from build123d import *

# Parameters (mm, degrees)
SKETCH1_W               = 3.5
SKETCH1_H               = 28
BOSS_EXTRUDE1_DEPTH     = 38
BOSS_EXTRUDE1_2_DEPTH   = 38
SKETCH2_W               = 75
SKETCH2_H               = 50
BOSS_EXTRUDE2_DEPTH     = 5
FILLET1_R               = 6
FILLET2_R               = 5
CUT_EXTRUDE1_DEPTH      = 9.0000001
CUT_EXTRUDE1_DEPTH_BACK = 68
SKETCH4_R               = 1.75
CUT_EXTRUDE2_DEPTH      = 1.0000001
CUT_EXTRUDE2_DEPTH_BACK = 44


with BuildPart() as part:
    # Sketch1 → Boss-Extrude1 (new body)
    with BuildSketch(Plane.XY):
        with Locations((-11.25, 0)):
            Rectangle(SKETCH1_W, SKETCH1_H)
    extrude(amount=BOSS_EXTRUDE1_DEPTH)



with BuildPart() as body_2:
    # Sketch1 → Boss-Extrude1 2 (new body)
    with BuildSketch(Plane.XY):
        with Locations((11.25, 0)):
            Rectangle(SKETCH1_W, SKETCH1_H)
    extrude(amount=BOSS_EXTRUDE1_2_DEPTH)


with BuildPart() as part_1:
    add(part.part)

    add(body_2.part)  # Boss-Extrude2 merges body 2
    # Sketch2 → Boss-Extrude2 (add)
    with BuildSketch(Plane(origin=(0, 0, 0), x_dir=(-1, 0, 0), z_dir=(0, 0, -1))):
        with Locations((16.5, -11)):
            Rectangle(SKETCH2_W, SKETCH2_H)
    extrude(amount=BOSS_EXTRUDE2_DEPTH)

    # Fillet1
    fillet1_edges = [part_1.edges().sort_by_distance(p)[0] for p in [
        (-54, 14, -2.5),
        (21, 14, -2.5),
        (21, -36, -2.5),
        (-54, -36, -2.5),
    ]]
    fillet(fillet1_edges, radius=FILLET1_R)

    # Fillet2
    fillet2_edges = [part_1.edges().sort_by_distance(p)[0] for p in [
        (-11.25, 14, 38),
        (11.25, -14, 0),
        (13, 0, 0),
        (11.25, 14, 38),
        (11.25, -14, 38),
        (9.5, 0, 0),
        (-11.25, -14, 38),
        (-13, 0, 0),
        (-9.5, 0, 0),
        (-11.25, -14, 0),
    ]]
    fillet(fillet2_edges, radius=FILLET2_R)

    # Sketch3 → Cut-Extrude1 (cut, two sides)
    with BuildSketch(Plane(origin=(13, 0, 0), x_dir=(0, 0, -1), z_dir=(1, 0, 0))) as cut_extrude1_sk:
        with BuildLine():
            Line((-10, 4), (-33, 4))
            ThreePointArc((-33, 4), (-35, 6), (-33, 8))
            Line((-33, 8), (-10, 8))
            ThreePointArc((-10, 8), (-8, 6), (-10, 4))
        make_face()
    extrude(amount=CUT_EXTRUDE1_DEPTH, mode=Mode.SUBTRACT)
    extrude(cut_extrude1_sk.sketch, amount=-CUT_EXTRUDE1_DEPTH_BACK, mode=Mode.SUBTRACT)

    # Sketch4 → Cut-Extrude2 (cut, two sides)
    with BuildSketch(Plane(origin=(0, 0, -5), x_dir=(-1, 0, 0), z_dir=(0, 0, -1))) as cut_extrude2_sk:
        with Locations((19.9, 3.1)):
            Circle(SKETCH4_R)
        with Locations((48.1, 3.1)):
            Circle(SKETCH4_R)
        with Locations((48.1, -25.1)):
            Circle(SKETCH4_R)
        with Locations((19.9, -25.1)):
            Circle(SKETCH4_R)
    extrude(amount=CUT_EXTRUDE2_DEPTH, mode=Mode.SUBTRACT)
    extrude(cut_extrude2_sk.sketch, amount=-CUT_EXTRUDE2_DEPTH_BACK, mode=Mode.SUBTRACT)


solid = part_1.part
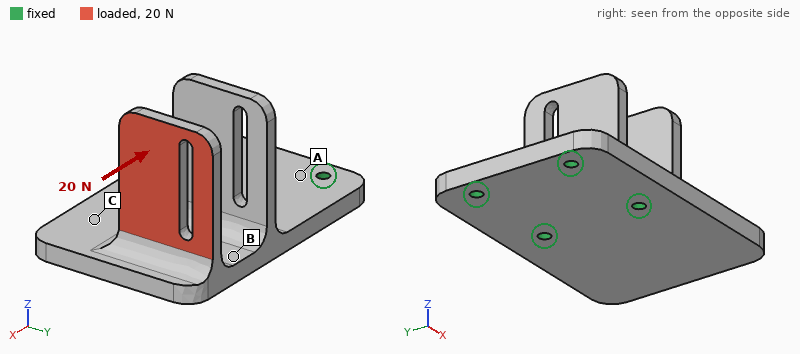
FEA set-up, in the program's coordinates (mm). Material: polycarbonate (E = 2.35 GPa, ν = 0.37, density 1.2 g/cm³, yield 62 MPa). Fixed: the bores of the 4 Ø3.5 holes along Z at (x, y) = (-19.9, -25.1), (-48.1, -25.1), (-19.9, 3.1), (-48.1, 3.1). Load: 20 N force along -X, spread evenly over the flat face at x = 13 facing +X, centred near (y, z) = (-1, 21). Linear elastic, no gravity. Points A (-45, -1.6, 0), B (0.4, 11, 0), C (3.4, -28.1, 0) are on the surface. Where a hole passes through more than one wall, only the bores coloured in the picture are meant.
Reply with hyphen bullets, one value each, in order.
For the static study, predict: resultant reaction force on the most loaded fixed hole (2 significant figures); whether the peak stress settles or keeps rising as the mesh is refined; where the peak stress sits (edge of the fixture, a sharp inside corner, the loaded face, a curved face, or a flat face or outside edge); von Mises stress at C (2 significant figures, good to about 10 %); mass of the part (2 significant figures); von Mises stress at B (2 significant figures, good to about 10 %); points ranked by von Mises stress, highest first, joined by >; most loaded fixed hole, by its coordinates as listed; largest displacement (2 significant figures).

- 14 N
- keeps rising
- edge of the fixture
- 1.3 MPa
- 31 g
- 2.8 MPa
- B > C > A
- (-19.9, 3.1)
- 1.00 mm
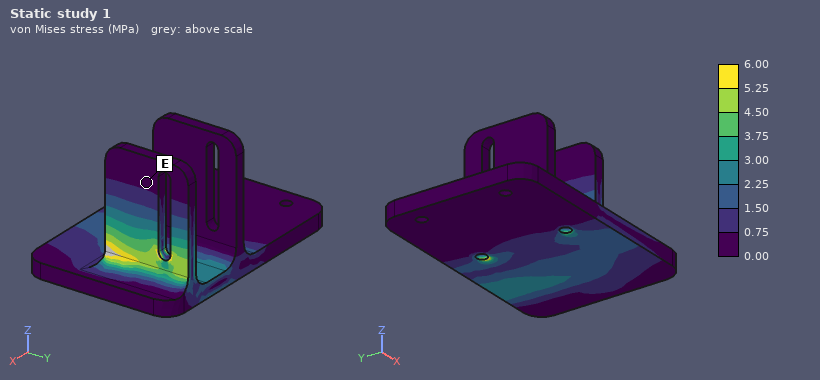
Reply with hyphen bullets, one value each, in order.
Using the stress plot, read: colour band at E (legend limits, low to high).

- 0.00 to 0.75 MPa
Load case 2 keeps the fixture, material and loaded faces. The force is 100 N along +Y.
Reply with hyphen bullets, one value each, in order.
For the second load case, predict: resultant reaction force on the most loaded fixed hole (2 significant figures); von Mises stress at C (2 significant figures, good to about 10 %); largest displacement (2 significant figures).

- 130 N
- 3.4 MPa
- 1.1 mm
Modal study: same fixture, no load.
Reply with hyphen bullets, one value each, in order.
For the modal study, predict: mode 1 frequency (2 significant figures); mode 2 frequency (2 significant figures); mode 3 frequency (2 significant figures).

- 390 Hz
- 600 Hz
- 810 Hz
